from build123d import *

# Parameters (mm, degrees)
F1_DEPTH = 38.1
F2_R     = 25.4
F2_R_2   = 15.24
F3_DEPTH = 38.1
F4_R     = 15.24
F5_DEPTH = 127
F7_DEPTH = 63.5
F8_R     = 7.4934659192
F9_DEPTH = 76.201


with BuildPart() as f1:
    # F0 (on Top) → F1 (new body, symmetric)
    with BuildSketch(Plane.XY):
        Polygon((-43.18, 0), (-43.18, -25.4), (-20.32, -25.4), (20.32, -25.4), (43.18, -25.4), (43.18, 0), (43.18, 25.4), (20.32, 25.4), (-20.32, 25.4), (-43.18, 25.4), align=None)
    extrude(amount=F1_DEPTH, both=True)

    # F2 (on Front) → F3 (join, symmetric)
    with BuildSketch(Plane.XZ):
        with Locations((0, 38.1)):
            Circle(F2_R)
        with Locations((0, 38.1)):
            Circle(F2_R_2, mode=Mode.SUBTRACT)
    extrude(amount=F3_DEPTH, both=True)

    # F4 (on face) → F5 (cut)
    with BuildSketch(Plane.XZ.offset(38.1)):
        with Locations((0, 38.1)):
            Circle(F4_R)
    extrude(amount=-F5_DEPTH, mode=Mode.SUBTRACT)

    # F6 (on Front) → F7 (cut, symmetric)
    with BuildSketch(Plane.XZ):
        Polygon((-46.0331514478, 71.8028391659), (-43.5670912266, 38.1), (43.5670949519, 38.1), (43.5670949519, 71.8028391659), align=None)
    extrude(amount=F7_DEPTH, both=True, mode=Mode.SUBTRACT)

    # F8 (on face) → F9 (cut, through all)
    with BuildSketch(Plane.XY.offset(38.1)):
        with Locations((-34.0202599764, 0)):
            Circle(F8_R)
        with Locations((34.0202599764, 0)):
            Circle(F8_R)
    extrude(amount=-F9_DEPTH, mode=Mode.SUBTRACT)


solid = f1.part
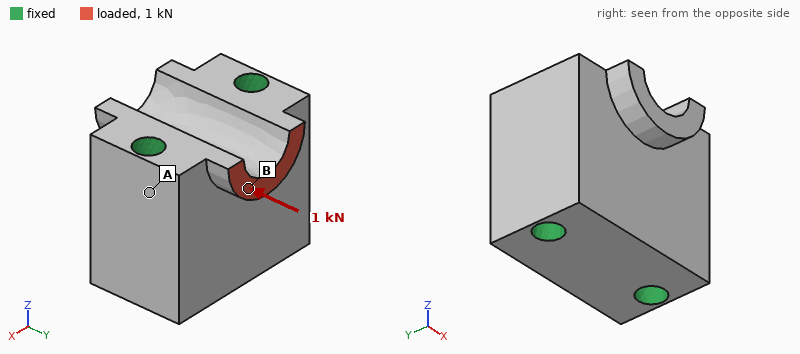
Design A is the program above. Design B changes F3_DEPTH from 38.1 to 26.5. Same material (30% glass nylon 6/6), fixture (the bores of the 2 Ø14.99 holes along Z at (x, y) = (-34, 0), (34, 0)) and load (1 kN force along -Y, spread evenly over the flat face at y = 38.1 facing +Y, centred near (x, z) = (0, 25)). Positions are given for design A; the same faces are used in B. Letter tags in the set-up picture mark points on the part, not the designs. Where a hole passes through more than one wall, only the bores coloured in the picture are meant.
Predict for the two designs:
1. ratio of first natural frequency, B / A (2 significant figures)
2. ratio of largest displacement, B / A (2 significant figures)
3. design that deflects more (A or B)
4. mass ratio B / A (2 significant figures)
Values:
1.0
0.79
A
0.95
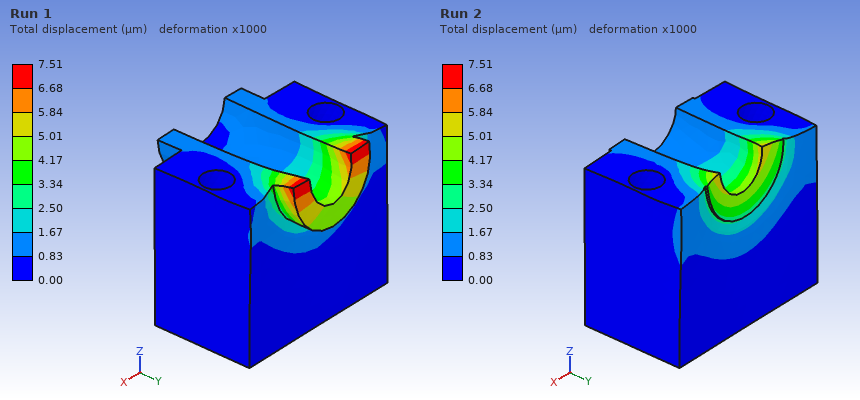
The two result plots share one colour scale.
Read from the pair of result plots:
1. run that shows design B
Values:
Run 2
